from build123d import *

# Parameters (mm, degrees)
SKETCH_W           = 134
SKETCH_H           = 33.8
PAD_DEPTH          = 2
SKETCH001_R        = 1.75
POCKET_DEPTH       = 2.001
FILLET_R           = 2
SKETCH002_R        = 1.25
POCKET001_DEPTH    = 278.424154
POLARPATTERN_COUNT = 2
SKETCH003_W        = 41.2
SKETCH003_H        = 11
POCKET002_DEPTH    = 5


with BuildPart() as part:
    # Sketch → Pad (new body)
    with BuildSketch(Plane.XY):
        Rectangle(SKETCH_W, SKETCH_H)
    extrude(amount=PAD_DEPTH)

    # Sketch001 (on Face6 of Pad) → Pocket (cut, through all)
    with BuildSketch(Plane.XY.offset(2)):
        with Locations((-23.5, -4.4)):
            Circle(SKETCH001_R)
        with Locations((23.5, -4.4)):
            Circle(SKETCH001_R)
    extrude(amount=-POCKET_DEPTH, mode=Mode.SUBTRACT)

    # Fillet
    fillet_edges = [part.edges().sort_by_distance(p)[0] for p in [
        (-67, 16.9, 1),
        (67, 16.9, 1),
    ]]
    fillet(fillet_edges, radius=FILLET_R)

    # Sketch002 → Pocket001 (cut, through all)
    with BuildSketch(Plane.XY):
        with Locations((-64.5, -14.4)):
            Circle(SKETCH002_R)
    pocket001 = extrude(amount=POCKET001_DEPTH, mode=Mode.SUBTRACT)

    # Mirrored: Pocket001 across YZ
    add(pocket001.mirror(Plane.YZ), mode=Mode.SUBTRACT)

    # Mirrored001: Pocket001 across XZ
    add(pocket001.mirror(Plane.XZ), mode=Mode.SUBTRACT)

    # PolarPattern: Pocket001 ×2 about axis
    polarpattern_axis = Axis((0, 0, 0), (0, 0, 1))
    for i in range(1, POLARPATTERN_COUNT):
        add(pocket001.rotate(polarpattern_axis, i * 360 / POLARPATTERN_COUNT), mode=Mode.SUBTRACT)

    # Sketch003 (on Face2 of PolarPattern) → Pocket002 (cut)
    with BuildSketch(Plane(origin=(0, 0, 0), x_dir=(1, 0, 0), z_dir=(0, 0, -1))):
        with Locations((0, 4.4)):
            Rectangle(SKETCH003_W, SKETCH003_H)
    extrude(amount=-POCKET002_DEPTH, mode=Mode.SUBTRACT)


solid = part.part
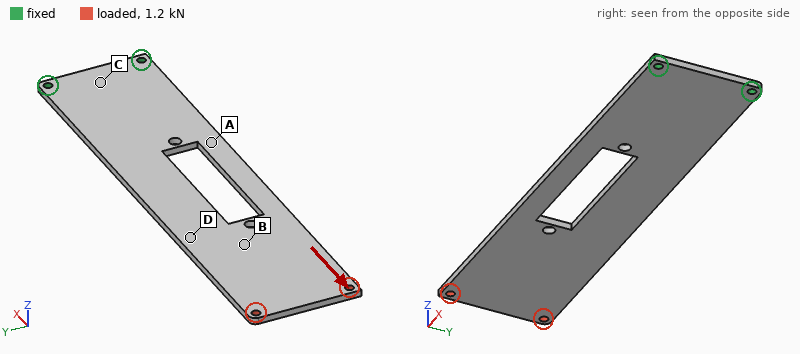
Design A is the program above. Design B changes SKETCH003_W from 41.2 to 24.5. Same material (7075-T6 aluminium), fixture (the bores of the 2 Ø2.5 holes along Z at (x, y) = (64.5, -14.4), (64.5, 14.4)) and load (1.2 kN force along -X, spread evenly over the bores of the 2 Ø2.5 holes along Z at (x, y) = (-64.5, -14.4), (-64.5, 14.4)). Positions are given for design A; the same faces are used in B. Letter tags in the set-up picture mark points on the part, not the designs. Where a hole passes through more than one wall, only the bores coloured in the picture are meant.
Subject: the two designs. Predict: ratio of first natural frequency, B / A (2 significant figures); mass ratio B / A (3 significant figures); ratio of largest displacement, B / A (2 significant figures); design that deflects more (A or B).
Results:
1.0
1.05
0.90
A
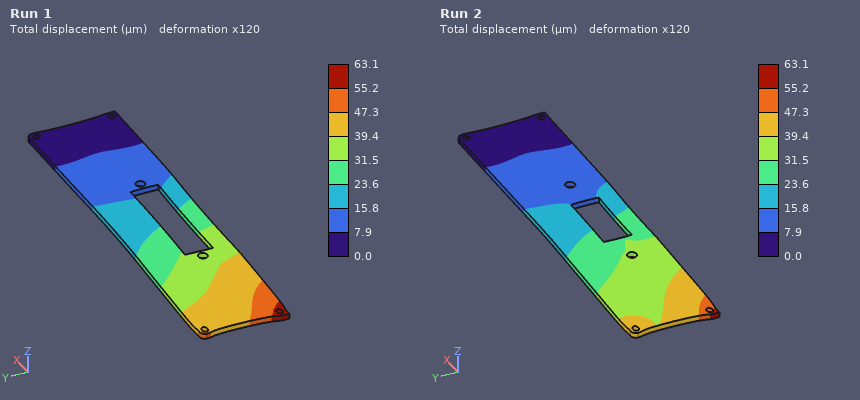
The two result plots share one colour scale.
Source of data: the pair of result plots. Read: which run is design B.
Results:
Run 2
